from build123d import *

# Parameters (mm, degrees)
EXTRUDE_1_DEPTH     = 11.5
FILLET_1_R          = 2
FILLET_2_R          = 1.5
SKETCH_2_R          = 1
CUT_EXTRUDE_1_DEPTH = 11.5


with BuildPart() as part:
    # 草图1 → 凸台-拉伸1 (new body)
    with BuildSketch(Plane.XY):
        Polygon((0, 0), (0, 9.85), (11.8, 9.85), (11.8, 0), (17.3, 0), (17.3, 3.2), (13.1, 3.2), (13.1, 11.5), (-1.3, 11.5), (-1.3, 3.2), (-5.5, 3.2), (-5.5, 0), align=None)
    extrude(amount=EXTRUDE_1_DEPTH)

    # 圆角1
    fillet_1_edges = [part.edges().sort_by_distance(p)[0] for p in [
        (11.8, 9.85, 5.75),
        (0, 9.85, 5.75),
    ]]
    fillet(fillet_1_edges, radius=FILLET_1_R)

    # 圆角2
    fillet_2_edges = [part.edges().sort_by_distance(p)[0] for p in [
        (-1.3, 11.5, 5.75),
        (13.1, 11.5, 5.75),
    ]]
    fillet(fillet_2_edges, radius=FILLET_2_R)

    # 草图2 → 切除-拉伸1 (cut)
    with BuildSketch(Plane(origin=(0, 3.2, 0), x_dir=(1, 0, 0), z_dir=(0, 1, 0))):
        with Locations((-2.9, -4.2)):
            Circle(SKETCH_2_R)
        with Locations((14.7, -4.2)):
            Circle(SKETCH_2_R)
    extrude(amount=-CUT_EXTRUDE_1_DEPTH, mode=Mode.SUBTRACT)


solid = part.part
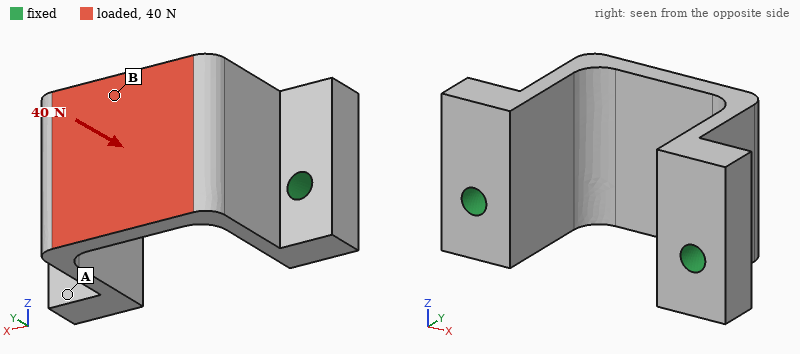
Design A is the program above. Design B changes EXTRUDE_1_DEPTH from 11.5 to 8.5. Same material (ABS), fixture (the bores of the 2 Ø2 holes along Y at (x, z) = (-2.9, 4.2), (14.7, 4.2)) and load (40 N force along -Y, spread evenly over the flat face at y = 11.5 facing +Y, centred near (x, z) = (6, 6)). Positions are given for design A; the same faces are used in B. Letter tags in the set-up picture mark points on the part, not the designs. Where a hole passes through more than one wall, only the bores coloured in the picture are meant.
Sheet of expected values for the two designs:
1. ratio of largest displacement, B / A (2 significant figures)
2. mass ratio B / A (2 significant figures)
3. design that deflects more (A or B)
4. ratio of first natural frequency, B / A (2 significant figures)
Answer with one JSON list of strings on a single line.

["1.1", "0.73", "B", "1.0"]
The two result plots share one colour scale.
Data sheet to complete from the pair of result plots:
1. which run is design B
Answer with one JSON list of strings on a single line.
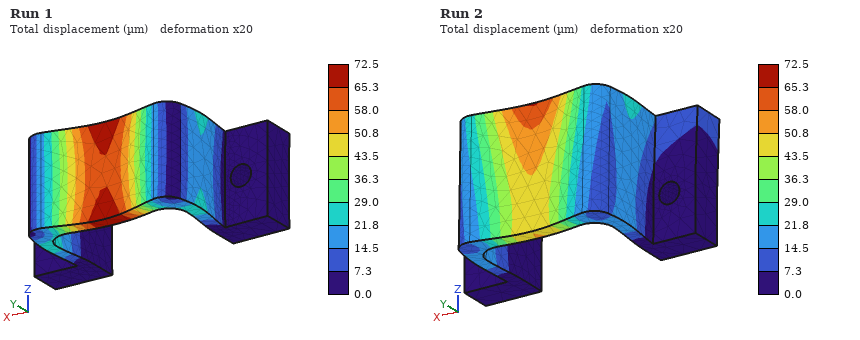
["Run 1"]
